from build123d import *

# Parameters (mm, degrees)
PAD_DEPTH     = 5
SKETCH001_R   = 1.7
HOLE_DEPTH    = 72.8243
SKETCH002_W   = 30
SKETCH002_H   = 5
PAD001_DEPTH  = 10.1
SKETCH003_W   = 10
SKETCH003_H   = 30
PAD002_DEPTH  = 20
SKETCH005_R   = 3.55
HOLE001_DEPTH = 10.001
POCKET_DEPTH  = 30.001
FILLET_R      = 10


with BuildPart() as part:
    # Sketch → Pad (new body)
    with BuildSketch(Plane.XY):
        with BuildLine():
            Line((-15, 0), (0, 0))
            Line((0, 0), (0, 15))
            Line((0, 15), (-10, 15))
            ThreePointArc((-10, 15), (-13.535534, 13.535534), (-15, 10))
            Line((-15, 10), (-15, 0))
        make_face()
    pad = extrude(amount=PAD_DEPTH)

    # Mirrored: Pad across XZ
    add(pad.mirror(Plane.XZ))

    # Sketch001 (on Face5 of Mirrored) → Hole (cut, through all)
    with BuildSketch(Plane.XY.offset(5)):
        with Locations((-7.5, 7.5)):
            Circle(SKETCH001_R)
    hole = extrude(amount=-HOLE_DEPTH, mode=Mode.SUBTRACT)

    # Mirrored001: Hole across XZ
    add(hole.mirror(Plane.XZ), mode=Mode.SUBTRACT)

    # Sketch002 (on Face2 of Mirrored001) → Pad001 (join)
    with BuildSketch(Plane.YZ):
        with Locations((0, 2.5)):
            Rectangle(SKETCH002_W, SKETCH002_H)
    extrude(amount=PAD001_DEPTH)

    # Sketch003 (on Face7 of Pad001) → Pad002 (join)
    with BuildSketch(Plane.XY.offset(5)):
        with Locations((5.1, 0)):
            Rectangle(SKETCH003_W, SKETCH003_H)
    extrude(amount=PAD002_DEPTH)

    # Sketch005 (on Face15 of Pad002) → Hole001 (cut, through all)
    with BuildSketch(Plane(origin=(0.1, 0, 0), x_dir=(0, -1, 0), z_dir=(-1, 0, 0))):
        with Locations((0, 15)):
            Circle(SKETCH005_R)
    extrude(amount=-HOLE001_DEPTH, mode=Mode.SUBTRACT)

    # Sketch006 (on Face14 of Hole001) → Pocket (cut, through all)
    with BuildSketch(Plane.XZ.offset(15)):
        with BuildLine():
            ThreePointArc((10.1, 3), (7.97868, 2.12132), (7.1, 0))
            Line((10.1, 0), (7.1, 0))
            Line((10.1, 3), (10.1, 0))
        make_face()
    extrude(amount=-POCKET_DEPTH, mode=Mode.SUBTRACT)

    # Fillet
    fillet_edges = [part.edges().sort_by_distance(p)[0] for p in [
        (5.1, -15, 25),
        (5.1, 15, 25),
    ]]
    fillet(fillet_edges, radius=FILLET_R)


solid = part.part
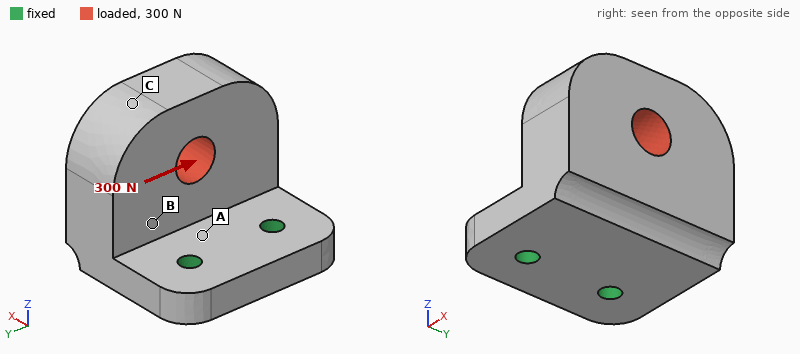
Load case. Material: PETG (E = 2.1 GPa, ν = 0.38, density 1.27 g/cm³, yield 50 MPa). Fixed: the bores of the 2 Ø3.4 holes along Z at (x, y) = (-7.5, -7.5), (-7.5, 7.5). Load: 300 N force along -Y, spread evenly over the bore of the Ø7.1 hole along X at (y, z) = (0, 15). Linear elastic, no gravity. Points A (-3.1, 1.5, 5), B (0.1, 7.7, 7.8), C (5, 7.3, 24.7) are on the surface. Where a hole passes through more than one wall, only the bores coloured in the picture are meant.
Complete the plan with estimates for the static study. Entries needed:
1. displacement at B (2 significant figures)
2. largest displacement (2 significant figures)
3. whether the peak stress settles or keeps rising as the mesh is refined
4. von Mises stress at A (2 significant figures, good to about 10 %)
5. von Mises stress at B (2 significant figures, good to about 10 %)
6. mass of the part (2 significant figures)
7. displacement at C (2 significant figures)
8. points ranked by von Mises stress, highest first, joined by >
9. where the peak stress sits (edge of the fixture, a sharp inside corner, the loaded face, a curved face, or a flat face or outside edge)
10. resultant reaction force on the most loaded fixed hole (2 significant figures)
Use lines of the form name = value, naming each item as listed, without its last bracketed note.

displacement at B = 0.14 mm
largest displacement = 0.35 mm
whether the peak stress settles or keeps rising as the mesh is refined = keeps rising
von Mises stress at A = 12 MPa
von Mises stress at B = 6.0 MPa
mass of the part = 11 g
displacement at C = 0.35 mm
points ranked by von Mises stress, highest first, joined by > = A > B > C
where the peak stress sits = edge of the fixture
resultant reaction force on the most loaded fixed hole = 320 N
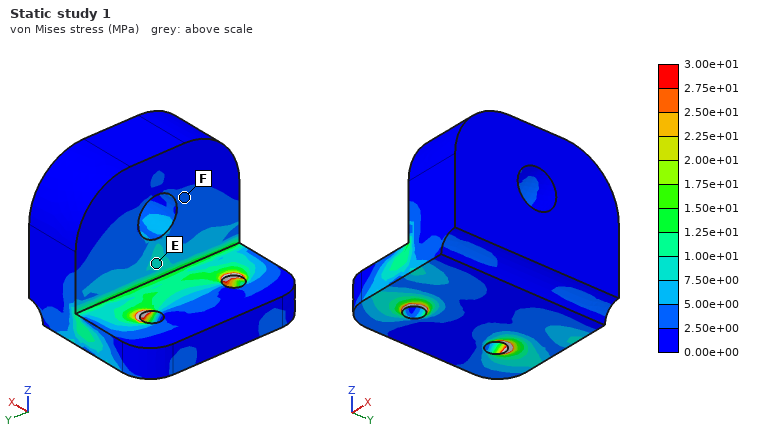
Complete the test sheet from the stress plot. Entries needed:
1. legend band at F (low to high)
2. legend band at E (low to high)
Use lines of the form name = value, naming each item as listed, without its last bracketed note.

legend band at F = 2.50e+00 to 5.00e+00 MPa
legend band at E = 7.50e+00 to 1.00e+01 MPa
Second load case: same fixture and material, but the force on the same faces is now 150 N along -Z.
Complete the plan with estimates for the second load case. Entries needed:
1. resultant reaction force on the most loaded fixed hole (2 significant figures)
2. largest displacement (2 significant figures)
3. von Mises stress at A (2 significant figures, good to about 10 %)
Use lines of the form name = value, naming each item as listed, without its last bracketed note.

resultant reaction force on the most loaded fixed hole = 75 N
largest displacement = 0.47 mm
von Mises stress at A = 7.3 MPa
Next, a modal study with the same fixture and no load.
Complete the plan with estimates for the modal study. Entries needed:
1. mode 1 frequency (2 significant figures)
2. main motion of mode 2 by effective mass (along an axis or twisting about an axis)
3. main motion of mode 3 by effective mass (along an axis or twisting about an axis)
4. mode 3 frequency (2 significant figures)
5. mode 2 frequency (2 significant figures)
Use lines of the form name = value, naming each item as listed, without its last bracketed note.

mode 1 frequency = 980 Hz
main motion of mode 2 by effective mass = along Y
main motion of mode 3 by effective mass = along Z
mode 3 frequency = 3900 Hz
mode 2 frequency = 1900 Hz
